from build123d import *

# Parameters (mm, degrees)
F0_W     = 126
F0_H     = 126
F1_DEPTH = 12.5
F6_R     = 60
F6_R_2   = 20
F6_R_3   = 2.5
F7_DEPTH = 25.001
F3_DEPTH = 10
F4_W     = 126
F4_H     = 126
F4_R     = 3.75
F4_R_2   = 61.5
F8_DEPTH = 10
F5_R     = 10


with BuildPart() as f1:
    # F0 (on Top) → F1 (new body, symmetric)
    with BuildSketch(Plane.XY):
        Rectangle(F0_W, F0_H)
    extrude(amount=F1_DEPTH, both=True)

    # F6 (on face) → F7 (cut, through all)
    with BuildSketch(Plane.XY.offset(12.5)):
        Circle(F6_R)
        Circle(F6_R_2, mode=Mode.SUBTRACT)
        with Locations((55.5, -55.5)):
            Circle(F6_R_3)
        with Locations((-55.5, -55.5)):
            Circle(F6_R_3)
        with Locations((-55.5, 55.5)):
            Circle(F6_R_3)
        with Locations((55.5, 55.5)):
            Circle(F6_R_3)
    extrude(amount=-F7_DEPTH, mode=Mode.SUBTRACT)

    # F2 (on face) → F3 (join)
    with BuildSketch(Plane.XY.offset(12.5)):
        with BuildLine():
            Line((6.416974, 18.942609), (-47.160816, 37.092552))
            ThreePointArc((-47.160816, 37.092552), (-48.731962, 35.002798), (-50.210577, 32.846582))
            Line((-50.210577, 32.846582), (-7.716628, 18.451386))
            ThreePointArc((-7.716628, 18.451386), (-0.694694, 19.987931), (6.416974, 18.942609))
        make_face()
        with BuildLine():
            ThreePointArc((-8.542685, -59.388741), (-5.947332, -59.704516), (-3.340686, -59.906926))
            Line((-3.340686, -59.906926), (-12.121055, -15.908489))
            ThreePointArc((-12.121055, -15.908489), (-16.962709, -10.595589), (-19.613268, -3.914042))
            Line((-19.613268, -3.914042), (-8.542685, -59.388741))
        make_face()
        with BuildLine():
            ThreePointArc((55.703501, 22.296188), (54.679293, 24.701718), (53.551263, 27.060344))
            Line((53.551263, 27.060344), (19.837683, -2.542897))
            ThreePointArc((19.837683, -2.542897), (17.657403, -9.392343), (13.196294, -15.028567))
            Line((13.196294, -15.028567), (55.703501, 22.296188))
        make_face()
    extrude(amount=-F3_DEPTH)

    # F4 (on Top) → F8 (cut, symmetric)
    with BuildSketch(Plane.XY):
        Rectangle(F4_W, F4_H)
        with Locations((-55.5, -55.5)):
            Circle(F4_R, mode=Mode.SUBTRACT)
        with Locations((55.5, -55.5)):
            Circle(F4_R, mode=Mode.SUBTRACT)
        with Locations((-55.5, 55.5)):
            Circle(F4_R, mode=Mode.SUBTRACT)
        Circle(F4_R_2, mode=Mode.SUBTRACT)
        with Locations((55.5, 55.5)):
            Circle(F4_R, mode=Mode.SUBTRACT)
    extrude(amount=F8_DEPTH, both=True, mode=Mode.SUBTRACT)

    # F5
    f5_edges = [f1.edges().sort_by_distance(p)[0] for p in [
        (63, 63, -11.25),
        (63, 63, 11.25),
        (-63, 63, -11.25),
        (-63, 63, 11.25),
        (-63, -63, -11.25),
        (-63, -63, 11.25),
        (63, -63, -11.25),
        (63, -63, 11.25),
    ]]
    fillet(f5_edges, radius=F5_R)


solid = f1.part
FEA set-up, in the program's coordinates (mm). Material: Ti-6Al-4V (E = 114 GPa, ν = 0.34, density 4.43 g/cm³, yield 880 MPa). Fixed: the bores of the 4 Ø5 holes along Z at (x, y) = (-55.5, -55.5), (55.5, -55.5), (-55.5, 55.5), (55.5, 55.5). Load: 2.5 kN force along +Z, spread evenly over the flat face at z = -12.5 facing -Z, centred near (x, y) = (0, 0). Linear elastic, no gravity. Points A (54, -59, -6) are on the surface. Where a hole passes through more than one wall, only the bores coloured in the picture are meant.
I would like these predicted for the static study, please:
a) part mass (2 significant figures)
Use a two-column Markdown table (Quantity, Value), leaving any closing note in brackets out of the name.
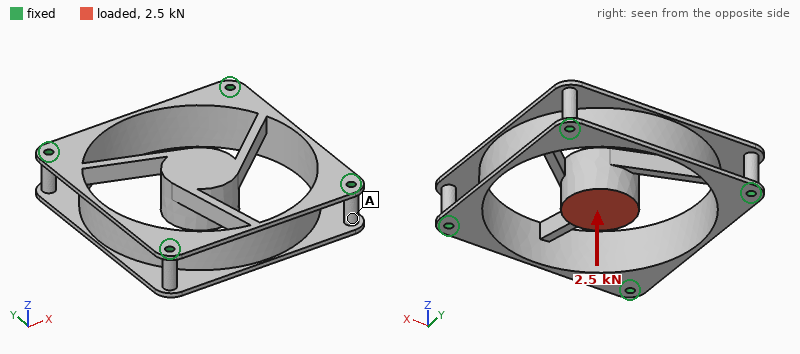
| Quantity | Value |
|---|---|
| part mass | 330 g |
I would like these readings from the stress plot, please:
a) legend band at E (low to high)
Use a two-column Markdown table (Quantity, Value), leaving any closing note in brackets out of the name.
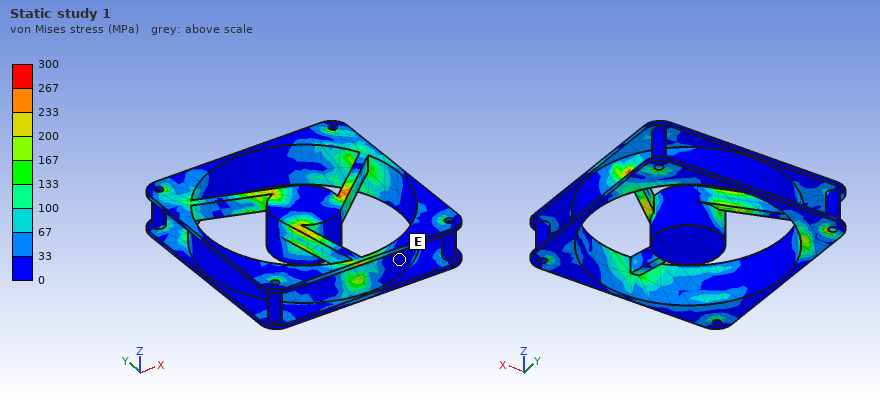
| Quantity | Value |
|---|---|
| legend band at E | 0 to 33 MPa |
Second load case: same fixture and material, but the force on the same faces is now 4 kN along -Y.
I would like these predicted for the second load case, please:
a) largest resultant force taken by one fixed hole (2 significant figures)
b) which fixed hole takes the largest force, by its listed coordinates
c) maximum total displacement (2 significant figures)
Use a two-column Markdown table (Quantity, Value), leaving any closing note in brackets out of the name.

| Quantity | Value |
|---|---|
| largest resultant force taken by one fixed hole | 3.3 kN |
| which fixed hole takes the largest force, by its listed coordinates | (-55.5, -55.5) |
| maximum total displacement | 0.52 mm |
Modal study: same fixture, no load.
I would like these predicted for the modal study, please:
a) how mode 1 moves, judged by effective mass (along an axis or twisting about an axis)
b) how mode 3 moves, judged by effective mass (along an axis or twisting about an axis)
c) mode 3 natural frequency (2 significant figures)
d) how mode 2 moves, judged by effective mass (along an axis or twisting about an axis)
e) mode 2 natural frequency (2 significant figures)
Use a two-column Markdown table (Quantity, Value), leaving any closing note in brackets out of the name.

| Quantity | Value |
|---|---|
| how mode 1 moves, judged by effective mass | along Z |
| how mode 3 moves, judged by effective mass | along X |
| mode 3 natural frequency | 2100 Hz |
| how mode 2 moves, judged by effective mass | along Y |
| mode 2 natural frequency | 1500 Hz |
